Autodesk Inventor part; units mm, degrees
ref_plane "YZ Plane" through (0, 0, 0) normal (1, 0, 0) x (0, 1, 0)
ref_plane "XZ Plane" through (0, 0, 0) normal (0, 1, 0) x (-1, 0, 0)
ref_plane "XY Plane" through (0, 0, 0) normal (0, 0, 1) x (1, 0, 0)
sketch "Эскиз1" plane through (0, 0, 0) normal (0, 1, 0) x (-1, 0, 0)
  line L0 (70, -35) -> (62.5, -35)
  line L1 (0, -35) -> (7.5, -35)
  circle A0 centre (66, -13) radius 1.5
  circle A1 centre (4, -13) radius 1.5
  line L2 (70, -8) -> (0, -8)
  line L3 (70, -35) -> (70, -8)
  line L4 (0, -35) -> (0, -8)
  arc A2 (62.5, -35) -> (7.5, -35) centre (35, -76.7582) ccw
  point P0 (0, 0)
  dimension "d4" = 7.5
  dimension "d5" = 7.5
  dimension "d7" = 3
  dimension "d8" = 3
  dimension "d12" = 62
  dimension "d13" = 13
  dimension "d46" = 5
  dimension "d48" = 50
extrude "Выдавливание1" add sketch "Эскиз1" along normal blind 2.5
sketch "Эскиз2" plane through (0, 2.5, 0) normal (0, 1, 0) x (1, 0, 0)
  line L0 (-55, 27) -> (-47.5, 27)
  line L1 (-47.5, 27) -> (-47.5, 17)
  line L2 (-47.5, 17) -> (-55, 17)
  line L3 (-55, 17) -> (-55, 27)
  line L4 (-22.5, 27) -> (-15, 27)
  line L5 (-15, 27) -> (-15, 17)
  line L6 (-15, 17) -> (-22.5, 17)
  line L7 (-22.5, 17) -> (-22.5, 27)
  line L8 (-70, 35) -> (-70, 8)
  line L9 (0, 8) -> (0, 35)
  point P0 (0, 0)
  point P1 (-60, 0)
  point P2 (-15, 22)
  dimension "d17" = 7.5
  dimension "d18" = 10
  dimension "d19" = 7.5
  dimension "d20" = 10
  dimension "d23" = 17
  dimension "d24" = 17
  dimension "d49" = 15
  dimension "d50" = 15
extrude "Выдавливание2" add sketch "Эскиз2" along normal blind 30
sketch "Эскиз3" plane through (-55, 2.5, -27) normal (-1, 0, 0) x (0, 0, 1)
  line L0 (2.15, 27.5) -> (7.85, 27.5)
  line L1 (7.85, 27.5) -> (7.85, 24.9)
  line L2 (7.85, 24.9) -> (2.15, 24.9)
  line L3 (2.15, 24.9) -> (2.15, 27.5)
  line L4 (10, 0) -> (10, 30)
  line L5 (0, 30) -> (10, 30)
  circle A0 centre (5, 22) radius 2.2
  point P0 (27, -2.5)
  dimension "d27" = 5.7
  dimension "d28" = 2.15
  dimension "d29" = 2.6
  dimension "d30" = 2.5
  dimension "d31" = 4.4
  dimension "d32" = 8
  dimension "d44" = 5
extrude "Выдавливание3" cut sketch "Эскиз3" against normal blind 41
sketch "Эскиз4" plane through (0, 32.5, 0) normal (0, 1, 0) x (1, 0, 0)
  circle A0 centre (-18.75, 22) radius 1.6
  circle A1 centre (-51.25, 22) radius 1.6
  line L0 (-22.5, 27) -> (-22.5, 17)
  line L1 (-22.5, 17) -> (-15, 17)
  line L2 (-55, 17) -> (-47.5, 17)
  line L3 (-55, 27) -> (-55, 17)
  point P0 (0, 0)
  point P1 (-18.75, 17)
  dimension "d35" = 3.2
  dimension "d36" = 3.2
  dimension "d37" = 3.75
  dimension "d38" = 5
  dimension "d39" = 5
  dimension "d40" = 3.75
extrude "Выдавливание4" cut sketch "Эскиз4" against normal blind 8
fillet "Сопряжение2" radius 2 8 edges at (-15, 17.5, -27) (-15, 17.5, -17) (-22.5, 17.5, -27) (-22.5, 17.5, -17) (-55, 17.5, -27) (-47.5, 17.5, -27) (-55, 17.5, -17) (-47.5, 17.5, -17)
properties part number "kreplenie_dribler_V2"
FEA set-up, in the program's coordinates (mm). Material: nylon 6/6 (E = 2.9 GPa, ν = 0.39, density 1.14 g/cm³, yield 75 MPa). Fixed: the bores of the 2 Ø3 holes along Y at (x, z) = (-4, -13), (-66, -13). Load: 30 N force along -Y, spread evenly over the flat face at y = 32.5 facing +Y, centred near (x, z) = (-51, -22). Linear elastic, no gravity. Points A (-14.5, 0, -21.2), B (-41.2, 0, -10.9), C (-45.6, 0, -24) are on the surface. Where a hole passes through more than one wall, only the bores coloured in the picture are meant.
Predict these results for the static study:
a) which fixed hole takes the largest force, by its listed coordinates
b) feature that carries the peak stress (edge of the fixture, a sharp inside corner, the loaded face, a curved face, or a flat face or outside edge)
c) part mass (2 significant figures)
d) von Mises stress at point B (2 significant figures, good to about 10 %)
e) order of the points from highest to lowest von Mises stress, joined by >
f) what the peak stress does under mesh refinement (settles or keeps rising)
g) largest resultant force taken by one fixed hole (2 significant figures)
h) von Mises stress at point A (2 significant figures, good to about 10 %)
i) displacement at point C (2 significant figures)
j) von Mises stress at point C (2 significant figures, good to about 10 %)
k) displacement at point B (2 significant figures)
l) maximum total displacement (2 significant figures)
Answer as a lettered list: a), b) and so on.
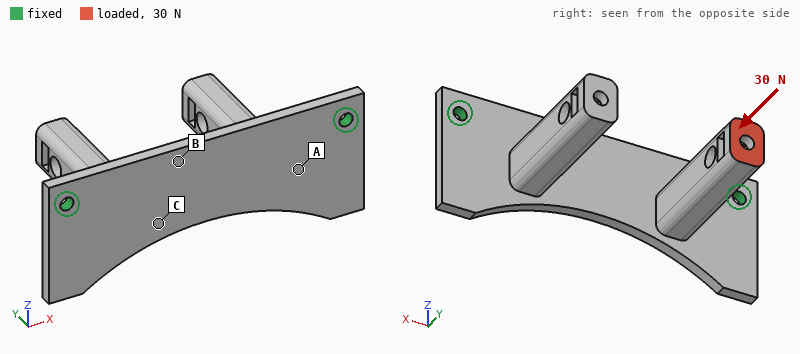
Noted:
a) (-66, -13)
b) edge of the fixture
c) 8.8 g
d) 4.3 MPa
e) C > B > A
f) keeps rising
g) 25 N
h) 1.8 MPa
i) 0.45 mm
j) 6.9 MPa
k) 0.22 mm
l) 0.92 mm
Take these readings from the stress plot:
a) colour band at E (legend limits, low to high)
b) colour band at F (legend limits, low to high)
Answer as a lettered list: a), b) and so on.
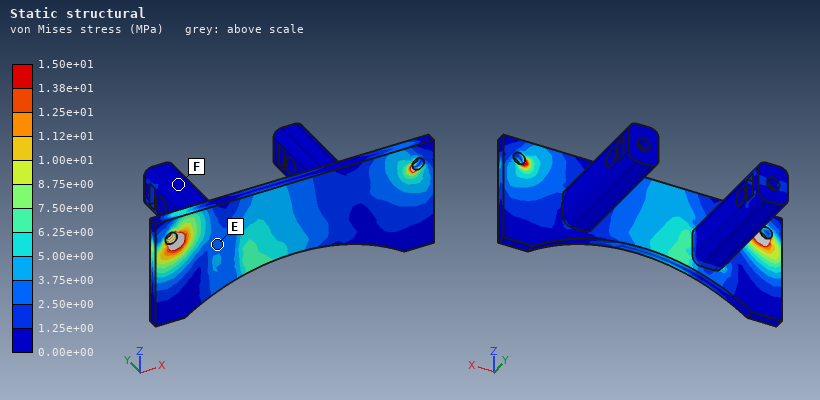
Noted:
a) 2.50e+00 to 3.75e+00 MPa
b) 0.00e+00 to 1.25e+00 MPa
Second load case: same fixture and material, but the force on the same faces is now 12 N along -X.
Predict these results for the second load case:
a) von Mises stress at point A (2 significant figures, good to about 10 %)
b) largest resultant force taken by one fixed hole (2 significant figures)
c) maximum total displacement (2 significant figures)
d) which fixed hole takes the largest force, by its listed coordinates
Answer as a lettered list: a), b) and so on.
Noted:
a) 1.5 MPa
b) 9.6 N
c) 0.88 mm
d) (-66, -13)
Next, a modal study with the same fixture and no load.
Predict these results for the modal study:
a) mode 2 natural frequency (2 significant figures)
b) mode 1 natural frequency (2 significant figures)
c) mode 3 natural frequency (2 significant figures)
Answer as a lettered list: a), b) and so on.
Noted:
a) 560 Hz
b) 400 Hz
c) 660 Hz
